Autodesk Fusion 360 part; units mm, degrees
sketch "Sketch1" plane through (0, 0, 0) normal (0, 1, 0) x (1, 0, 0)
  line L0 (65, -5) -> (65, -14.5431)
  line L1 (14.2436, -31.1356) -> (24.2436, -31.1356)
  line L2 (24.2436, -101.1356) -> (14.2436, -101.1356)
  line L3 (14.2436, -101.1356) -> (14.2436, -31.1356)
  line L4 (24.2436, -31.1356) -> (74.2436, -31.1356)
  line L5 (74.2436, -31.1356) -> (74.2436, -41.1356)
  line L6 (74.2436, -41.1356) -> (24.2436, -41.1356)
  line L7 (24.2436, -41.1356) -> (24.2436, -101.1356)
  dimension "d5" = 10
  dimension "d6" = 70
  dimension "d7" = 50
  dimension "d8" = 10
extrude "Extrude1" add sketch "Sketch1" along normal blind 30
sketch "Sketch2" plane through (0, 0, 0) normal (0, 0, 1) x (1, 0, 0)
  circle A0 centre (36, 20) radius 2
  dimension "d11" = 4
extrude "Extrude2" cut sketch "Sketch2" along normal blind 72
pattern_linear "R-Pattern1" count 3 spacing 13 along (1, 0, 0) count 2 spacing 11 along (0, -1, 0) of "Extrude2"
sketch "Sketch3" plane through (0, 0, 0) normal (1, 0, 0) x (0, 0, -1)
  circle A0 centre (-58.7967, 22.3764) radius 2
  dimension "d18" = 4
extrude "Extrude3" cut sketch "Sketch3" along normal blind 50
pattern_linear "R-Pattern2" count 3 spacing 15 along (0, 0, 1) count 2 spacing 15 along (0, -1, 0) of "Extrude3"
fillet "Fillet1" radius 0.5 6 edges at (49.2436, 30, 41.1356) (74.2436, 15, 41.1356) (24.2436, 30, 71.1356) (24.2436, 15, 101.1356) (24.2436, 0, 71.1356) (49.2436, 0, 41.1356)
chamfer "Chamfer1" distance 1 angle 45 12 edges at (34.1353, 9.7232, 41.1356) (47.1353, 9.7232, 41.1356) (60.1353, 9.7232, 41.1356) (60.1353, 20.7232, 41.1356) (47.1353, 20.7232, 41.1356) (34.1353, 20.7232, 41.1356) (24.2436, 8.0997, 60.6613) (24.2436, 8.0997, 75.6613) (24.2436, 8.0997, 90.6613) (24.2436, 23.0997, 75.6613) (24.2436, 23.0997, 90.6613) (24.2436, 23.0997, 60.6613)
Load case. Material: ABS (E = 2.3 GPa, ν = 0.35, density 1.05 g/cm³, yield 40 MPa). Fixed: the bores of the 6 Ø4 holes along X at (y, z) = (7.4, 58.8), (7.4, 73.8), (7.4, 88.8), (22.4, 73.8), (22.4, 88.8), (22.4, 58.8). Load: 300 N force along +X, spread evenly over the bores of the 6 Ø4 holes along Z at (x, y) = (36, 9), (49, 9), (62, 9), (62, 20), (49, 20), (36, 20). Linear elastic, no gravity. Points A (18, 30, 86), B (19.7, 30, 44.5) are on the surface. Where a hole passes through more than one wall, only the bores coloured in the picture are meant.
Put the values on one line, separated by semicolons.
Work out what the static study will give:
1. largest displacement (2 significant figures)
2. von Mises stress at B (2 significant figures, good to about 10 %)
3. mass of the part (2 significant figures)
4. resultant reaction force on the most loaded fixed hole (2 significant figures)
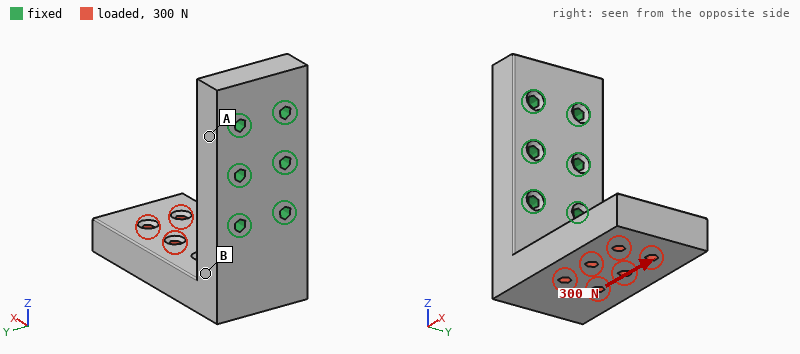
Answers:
0.91 mm; 3.7 MPa; 36 g; 200 N
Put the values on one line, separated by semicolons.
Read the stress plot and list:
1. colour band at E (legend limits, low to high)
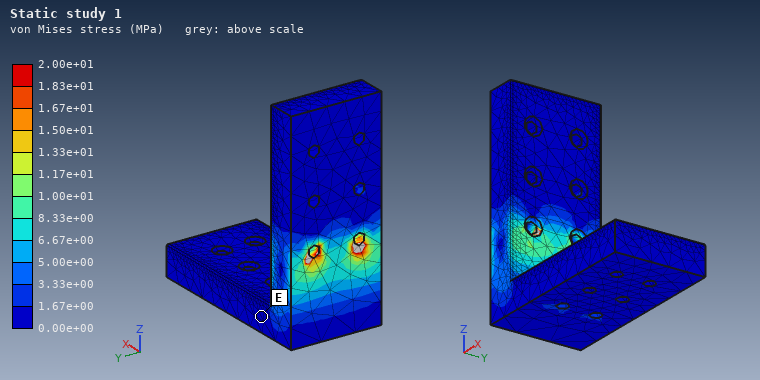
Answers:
0.00e+00 to 1.67e+00 MPa
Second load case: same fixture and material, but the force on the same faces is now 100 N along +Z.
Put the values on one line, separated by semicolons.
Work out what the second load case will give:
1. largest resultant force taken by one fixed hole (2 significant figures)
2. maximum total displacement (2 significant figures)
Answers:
48 N; 0.98 mm
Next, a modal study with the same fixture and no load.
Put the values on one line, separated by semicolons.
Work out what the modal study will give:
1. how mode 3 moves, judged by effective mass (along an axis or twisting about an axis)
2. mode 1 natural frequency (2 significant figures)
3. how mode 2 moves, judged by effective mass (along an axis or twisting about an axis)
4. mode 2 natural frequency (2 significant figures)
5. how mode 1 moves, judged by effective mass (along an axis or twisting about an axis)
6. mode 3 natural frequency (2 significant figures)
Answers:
along X; 490 Hz; along Y; 760 Hz; along Z; 1700 Hz
